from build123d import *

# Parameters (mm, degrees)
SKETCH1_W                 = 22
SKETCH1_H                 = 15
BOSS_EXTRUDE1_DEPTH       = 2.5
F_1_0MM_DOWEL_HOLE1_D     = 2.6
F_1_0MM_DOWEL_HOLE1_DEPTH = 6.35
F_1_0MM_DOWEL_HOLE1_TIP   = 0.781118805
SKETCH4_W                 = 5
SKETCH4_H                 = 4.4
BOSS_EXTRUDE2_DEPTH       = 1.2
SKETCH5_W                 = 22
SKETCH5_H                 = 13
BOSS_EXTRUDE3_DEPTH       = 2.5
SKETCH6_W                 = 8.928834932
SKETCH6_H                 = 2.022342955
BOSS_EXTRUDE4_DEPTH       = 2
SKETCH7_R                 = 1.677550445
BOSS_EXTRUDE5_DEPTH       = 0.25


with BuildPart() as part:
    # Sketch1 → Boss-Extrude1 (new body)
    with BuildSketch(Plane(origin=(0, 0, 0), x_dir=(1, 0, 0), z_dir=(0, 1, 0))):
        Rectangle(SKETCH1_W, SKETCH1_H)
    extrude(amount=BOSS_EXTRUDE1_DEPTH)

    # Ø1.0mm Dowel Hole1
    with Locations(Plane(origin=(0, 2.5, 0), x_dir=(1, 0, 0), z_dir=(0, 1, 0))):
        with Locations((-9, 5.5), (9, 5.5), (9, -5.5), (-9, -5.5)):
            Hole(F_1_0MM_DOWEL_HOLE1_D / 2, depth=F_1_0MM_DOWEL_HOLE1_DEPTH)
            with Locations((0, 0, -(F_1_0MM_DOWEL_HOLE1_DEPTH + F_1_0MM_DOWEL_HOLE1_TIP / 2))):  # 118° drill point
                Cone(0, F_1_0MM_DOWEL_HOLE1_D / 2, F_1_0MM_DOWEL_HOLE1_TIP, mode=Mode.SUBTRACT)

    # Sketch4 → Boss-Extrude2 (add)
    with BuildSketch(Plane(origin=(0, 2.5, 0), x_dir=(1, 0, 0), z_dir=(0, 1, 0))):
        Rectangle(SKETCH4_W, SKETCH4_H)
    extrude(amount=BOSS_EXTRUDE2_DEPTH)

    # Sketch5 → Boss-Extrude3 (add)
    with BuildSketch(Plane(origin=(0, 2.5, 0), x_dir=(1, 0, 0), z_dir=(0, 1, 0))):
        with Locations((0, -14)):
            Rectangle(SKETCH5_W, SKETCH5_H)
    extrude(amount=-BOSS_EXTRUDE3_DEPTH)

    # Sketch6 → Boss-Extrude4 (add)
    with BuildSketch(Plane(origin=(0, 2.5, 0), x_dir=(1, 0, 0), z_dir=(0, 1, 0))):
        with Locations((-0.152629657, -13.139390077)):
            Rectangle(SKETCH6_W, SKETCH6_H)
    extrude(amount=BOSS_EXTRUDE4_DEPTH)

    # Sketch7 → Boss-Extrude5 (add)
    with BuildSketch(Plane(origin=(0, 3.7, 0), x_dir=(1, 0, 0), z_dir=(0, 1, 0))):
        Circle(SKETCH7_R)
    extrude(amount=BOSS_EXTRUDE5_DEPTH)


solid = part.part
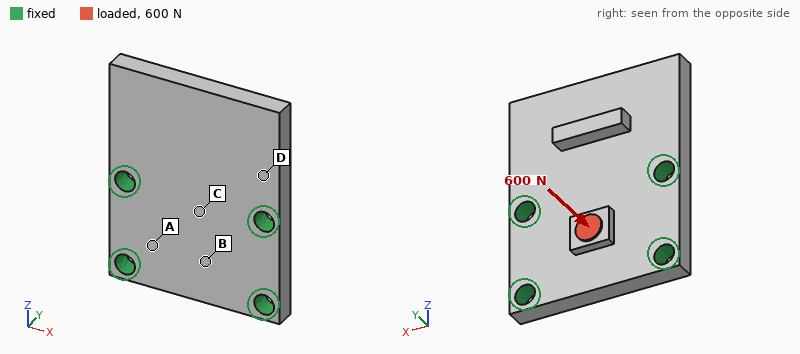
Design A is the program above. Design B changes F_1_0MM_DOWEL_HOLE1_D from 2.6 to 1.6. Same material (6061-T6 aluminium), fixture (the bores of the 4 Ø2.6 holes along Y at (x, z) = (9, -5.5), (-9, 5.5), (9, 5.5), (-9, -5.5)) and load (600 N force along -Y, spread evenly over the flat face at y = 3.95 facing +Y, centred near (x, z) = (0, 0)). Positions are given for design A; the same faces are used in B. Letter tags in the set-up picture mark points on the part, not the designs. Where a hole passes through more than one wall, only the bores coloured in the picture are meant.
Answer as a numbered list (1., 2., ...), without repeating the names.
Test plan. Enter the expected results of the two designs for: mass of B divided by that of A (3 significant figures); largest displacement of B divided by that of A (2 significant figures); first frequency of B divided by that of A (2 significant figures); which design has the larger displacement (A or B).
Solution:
1. 1.02
2. 1.2
3. 0.91
4. B
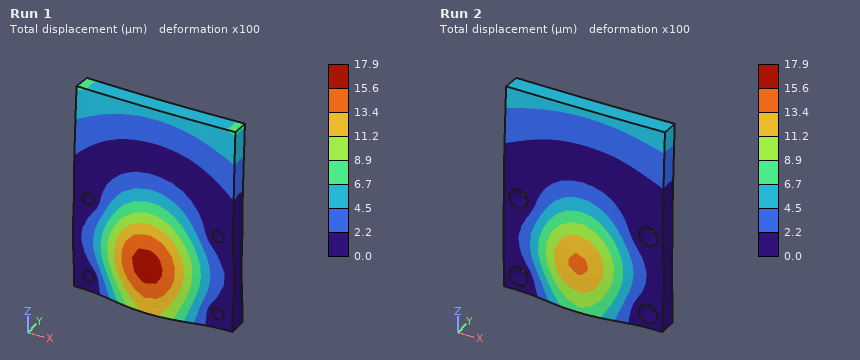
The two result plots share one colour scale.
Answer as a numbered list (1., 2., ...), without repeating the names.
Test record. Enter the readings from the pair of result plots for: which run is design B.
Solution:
1. Run 1
